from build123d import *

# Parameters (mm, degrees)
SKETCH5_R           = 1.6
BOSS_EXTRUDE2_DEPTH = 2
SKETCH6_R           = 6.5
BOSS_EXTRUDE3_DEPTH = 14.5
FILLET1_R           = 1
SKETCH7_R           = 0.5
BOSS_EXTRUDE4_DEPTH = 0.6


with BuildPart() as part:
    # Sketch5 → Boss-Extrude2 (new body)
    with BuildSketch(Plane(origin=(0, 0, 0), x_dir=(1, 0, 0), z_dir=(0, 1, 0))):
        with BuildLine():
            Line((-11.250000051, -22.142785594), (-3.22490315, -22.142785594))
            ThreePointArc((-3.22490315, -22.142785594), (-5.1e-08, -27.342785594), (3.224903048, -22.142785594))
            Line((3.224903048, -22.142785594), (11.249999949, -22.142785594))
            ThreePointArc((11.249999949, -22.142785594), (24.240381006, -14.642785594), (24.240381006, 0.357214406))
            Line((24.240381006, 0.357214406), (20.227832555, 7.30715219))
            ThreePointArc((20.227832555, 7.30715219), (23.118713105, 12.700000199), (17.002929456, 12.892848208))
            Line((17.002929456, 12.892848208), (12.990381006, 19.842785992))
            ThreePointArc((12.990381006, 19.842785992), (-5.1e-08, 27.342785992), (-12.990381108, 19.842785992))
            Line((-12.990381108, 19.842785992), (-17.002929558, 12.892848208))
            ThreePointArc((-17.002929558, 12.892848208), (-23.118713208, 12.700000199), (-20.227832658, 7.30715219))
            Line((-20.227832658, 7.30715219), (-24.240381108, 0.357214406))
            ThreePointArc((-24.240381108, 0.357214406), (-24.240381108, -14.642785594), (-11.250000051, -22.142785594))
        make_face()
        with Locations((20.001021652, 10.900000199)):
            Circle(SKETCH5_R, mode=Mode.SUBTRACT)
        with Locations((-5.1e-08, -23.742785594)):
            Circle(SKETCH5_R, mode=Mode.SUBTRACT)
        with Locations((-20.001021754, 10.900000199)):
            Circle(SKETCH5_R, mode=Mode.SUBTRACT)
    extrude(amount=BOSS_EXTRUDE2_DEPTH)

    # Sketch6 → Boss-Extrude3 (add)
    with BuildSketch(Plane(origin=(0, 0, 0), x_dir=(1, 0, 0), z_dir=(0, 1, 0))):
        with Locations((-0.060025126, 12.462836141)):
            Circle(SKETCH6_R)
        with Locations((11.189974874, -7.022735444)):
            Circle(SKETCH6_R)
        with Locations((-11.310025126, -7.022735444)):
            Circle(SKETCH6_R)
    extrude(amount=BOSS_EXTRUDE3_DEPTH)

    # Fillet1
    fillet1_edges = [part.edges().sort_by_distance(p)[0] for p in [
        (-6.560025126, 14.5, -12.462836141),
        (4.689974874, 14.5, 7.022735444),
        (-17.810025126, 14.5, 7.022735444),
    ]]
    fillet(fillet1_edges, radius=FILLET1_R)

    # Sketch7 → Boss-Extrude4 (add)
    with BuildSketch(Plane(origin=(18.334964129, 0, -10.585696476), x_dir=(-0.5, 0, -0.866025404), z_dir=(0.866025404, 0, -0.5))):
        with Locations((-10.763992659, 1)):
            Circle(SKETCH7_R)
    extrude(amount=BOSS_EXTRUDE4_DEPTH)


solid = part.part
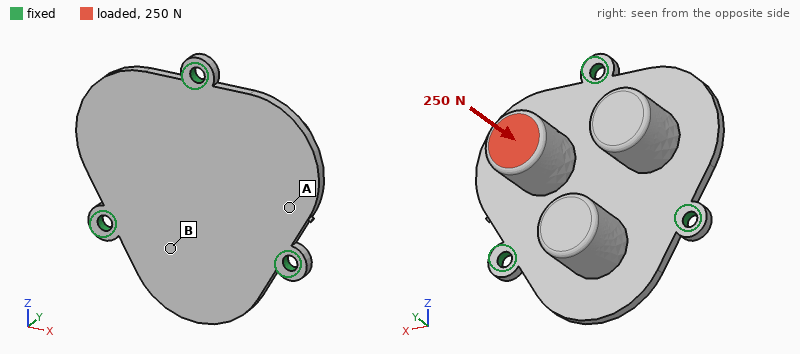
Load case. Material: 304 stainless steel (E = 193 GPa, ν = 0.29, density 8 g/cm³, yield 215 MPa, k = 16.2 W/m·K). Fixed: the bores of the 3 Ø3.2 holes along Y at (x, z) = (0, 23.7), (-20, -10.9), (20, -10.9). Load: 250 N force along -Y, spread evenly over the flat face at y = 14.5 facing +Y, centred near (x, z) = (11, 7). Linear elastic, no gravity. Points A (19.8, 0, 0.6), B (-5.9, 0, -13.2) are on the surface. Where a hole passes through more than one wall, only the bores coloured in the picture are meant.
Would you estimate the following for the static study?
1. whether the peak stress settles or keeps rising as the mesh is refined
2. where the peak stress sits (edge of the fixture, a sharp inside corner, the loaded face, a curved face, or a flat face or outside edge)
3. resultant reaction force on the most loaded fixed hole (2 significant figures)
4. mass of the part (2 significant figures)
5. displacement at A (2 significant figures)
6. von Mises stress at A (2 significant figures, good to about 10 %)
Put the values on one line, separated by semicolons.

keeps rising; edge of the fixture; 130 N; 72 g; 19 µm; 36 MPa
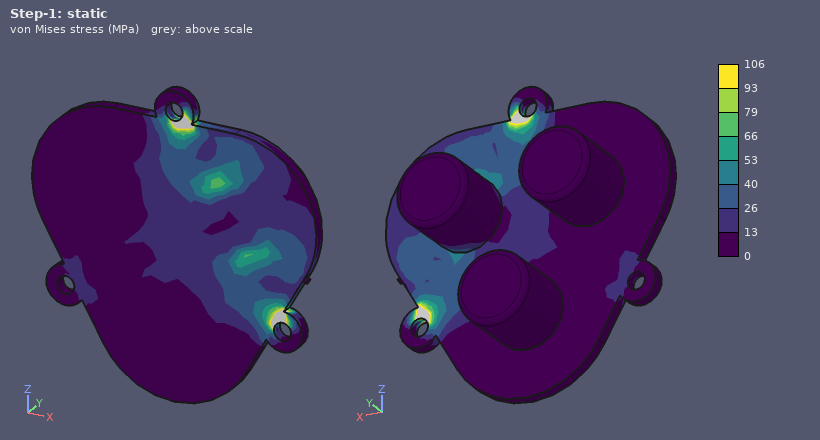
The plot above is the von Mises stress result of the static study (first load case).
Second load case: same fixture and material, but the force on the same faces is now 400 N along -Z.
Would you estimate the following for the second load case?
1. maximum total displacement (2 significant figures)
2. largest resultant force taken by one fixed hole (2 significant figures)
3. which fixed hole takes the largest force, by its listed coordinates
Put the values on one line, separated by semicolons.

60 µm; 260 N; (0, 23.7)
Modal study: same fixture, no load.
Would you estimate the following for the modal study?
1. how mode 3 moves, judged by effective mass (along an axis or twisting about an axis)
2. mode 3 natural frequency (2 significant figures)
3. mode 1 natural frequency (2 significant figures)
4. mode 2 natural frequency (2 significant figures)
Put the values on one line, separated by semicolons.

along Y; 3500 Hz; 3000 Hz; 3000 Hz
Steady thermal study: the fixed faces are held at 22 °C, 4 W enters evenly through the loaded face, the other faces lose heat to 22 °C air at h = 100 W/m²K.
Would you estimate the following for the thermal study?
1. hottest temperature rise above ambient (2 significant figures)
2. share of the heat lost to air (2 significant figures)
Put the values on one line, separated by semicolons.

38 K; 86 %
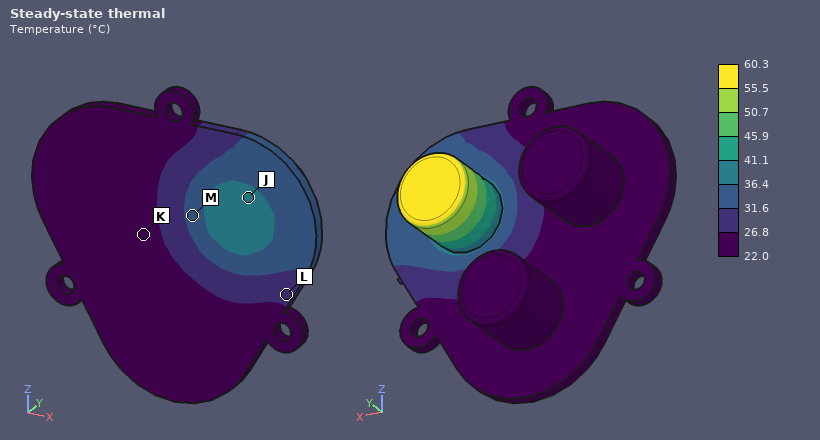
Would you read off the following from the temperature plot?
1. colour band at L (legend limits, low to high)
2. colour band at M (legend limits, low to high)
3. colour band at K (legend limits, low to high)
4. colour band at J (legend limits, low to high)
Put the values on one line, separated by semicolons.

26.8 to 31.6 °C; 31.6 to 36.4 °C; 22.0 to 26.8 °C; 36.4 to 41.1 °C
